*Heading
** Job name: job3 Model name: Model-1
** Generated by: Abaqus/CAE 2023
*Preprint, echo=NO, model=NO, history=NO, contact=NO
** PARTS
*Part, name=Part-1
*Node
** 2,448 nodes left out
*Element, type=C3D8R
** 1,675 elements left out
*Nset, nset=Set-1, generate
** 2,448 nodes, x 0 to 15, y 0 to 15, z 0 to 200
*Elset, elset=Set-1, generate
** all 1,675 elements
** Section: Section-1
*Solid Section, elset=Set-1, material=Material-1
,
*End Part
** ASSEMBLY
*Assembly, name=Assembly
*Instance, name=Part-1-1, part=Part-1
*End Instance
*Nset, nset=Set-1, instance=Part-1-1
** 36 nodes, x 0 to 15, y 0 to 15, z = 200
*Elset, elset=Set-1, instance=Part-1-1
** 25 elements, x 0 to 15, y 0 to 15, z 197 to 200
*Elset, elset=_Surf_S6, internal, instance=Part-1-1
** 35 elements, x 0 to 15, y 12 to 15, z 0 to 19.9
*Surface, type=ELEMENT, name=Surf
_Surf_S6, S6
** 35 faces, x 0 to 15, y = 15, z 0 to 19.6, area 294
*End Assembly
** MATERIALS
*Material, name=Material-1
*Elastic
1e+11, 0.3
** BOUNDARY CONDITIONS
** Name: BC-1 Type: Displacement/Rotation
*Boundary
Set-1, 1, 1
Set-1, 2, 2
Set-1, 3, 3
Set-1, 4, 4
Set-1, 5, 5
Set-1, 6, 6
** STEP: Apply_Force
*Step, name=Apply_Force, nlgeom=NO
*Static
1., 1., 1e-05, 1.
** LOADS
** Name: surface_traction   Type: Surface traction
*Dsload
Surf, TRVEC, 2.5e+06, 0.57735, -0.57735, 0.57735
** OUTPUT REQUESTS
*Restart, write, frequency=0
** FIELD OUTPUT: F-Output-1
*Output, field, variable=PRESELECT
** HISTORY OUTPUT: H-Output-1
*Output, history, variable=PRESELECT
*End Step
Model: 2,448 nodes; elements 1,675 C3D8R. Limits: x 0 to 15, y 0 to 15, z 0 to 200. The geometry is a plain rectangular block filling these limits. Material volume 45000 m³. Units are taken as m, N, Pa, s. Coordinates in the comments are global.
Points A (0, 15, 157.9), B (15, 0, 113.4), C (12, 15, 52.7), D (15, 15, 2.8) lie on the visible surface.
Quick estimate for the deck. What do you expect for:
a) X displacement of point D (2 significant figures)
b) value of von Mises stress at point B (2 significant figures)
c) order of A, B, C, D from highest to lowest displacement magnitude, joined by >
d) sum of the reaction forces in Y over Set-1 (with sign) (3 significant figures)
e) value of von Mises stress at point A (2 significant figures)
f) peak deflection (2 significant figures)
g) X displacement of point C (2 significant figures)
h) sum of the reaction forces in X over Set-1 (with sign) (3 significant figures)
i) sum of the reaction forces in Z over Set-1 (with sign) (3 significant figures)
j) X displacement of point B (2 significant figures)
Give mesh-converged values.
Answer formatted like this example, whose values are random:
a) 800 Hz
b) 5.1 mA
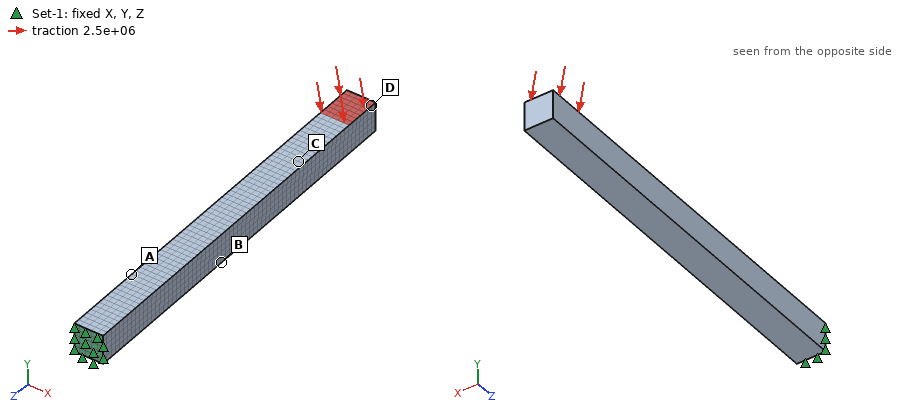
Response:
a) 2.4 m
b) 1.5e+08 Pa
c) D > C > B > A
d) 4.24e+08 N
e) 2.2e+08 Pa
f) 3.4 m
g) 1.6 m
h) -4.24e+08 N
i) -4.24e+08 N
j) 0.60 m
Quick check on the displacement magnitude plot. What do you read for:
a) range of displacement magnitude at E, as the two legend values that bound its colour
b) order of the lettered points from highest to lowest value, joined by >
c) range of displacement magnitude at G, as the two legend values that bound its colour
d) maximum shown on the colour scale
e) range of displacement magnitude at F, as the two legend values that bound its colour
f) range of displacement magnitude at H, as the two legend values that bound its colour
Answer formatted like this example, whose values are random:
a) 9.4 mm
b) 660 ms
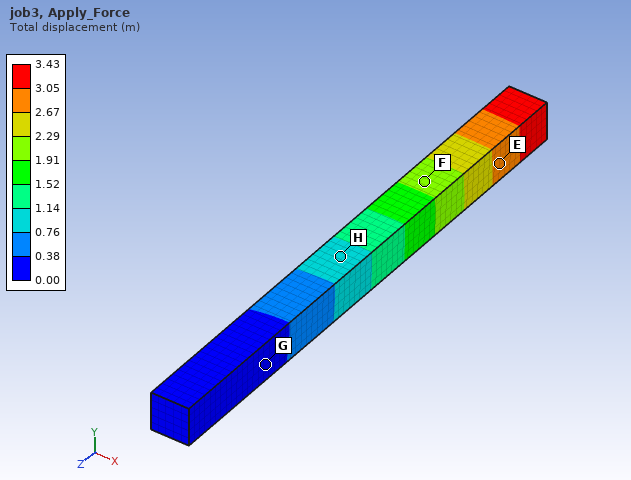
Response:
a) 2.67 to 3.05 m
b) E > F > H > G
c) 0.00 to 0.38 m
d) 3.43 m
e) 1.91 to 2.29 m
f) 0.76 to 1.14 m
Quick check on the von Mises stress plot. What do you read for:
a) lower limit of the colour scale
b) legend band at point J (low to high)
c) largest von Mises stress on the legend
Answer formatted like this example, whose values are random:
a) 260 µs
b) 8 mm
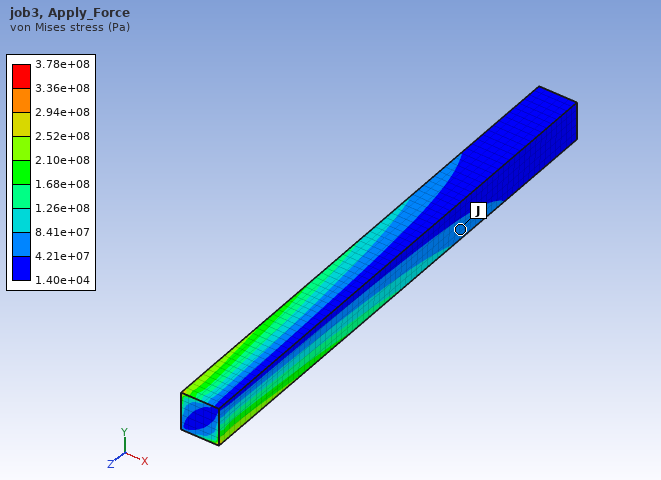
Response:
a) 1.40e+04 Pa
b) 4.21e+07 to 8.41e+07 Pa
c) 3.78e+08 Pa
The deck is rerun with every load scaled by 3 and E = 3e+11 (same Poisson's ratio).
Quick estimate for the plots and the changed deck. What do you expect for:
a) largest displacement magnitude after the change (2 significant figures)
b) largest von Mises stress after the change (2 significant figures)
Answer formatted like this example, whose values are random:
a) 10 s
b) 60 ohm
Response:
a) 3.4 m
b) 1.1e+09 Pa
